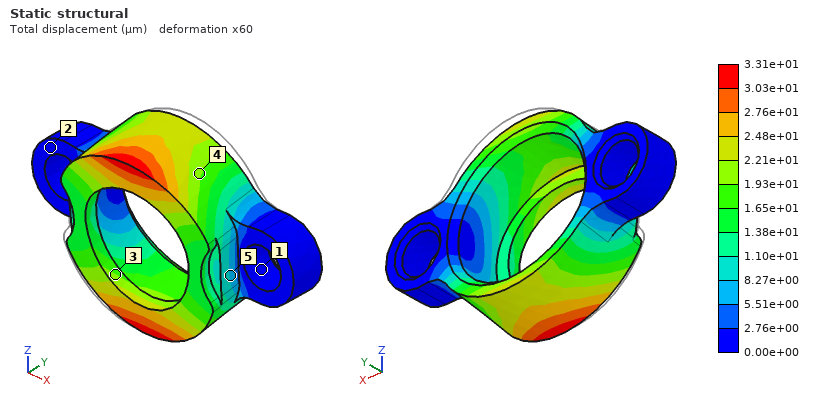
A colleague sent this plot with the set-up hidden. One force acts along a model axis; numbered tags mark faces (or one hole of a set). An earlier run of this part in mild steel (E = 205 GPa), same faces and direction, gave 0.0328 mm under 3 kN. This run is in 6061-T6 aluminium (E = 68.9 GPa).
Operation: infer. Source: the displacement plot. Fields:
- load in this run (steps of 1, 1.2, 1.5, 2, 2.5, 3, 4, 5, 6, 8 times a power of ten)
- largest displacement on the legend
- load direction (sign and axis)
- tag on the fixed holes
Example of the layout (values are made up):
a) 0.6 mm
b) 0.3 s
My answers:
a) 1 kN
b) 3.31e+01 µm
c) -Z
d) 1
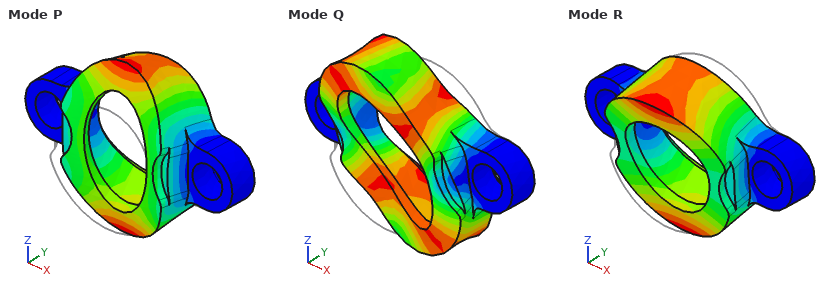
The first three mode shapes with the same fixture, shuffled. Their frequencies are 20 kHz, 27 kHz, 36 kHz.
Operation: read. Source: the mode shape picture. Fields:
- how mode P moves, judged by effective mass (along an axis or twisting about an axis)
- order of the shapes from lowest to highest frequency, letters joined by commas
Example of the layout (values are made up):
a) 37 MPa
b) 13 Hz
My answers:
a) along Y
b) R, P, Q
